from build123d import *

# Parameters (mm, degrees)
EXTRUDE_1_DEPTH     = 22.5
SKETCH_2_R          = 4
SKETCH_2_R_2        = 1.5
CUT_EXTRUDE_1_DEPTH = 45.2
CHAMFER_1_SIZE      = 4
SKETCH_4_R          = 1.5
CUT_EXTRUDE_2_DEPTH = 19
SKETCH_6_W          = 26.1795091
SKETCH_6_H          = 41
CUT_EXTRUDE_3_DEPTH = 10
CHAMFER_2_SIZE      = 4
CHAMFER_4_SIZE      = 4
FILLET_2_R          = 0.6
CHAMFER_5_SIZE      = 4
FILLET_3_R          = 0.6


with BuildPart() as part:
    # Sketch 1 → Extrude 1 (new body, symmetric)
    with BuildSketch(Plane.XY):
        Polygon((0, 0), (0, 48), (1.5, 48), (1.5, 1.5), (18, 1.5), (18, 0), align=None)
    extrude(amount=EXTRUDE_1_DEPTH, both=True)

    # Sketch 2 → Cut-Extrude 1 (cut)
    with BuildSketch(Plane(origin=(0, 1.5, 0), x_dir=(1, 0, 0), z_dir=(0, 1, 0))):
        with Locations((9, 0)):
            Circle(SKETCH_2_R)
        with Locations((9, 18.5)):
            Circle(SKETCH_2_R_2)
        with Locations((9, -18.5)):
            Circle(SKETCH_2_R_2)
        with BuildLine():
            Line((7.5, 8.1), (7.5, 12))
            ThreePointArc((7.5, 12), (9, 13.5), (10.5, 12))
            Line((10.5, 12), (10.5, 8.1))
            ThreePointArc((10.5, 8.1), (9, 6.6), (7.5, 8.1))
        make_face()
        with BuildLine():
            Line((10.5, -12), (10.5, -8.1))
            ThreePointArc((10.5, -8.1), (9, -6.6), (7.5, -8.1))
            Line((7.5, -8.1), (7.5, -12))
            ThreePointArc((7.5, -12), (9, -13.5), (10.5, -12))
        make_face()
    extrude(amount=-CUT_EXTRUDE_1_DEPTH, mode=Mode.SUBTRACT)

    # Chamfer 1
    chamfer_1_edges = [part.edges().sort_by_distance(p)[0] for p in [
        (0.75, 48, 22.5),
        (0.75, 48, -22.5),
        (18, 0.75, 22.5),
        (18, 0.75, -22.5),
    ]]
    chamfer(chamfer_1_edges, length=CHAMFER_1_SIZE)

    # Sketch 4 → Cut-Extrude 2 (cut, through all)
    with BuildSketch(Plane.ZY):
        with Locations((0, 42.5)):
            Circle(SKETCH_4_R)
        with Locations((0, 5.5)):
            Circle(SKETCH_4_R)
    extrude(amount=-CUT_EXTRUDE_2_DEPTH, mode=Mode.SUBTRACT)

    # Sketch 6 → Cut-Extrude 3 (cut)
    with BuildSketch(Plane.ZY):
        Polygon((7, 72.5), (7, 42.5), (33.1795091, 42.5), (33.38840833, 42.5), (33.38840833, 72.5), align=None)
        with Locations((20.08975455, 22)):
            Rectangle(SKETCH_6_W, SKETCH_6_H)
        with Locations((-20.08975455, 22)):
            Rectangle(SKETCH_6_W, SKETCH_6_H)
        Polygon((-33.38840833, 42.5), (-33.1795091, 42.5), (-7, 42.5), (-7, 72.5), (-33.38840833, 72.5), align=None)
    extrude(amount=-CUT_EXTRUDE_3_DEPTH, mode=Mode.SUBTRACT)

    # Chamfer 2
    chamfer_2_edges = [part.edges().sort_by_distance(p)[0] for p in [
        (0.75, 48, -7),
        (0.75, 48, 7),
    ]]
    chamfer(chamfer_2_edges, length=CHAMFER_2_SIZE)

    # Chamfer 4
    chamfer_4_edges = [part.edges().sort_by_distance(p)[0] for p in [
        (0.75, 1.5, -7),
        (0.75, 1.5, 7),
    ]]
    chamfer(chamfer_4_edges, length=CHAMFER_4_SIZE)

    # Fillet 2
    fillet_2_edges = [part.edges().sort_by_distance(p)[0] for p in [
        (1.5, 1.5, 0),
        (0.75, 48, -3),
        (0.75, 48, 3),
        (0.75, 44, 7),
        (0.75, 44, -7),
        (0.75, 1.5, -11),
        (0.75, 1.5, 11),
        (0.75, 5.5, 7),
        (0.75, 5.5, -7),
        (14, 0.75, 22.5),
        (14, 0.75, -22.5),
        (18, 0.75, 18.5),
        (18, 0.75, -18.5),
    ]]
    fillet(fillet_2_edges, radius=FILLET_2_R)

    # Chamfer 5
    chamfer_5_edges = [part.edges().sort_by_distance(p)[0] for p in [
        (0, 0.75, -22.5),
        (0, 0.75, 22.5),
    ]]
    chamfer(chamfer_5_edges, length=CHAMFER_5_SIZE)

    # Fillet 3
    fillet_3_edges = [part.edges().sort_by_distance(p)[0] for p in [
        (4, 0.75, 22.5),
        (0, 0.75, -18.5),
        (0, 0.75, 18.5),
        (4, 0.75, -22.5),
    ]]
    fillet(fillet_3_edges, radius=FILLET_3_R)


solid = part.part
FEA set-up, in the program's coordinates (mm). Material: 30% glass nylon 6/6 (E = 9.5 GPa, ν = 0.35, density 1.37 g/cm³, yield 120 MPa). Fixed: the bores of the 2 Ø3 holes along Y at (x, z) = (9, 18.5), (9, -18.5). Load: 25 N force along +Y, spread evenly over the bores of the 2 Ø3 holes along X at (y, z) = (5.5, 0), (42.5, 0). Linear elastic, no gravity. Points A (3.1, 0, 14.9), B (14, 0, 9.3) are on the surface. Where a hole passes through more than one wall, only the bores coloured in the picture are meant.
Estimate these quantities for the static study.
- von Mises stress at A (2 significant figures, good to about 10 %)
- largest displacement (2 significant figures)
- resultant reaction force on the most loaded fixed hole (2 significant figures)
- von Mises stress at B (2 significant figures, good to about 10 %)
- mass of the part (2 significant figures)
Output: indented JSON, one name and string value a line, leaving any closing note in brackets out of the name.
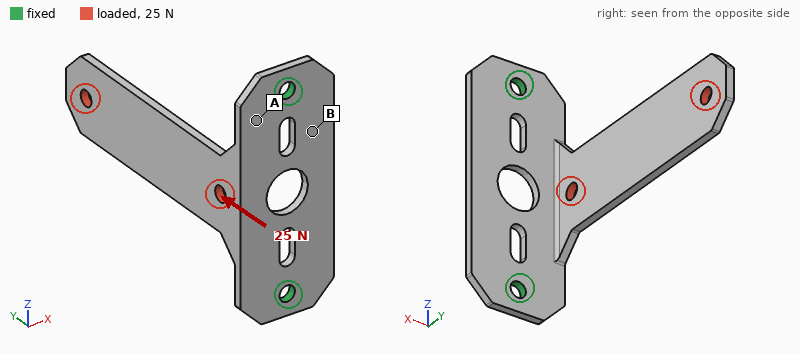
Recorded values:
{
  "von Mises stress at A": "11 MPa",
  "largest displacement": "0.76 mm",
  "resultant reaction force on the most loaded fixed hole": "15 N",
  "von Mises stress at B": "3.3 MPa",
  "mass of the part": "2.7 g"
}
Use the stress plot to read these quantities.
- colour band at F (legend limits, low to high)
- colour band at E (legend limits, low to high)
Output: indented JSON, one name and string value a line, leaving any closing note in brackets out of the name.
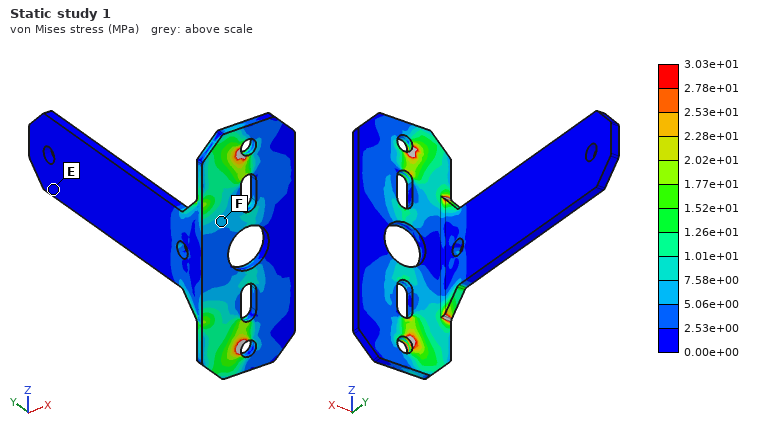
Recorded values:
{
  "colour band at F": "5.06e+00 to 7.58e+00 MPa",
  "colour band at E": "0.00e+00 to 2.53e+00 MPa"
}
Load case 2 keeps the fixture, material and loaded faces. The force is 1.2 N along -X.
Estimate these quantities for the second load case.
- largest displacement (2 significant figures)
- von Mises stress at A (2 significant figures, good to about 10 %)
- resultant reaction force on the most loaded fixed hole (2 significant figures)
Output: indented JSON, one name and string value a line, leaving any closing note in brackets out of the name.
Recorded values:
{
  "largest displacement": "0.66 mm",
  "von Mises stress at A": "2.2 MPa",
  "resultant reaction force on the most loaded fixed hole": "0.69 N"
}
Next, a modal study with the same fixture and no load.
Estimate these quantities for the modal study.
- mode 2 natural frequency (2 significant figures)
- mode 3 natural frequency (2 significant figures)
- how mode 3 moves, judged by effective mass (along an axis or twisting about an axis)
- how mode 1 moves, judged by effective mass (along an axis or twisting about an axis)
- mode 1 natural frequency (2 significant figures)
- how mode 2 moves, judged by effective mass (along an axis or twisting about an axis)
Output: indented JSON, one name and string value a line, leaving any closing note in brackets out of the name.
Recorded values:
{
  "mode 2 natural frequency": "1000 Hz",
  "mode 3 natural frequency": "1500 Hz",
  "how mode 3 moves, judged by effective mass": "along Y",
  "how mode 1 moves, judged by effective mass": "along X",
  "mode 1 natural frequency": "250 Hz",
  "how mode 2 moves, judged by effective mass": "along Z"
}
